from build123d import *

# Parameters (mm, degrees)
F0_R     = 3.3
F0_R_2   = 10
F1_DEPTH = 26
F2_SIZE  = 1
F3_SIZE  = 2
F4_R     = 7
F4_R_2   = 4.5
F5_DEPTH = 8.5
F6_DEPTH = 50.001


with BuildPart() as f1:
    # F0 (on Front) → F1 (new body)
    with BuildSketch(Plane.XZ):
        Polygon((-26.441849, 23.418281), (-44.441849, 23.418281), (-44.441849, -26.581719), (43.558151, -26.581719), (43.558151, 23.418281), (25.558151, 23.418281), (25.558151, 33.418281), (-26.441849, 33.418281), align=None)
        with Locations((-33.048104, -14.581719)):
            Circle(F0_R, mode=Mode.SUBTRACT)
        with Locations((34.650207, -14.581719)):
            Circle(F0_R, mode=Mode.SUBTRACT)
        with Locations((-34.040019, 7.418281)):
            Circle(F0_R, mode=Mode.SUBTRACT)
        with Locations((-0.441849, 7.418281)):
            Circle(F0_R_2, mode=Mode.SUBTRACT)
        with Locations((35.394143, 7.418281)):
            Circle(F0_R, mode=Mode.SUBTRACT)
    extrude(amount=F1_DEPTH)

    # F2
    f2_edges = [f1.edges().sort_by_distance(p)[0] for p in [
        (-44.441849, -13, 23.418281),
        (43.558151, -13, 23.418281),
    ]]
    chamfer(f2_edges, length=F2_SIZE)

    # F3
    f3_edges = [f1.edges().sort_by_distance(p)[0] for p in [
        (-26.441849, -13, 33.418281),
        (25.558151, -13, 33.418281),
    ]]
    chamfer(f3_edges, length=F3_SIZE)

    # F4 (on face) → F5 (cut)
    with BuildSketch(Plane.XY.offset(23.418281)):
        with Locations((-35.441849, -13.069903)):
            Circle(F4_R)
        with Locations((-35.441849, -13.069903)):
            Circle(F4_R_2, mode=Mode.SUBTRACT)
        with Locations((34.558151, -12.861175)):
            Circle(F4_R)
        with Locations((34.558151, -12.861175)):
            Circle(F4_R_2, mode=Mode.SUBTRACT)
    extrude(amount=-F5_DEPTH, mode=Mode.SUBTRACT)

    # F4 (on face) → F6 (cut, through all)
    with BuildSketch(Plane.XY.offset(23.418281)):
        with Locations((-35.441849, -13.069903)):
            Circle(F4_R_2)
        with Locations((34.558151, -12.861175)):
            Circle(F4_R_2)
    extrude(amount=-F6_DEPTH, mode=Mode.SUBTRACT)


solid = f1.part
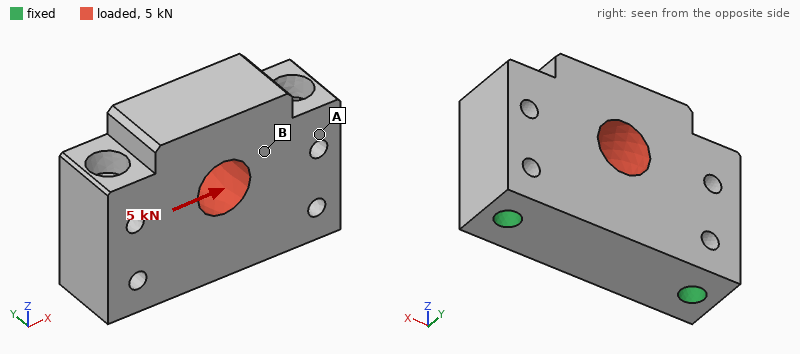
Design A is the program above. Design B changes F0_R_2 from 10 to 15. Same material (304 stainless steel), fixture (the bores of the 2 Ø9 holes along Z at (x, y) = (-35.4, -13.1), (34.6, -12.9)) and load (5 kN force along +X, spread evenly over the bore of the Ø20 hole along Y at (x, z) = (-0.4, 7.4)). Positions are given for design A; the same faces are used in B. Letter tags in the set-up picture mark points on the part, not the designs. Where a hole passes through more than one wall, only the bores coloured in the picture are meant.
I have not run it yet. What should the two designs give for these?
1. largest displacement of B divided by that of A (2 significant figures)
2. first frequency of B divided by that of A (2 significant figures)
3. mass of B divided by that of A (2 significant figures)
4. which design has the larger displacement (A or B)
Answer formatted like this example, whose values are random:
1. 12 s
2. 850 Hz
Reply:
1. 1.3
2. 1.0
3. 0.91
4. B
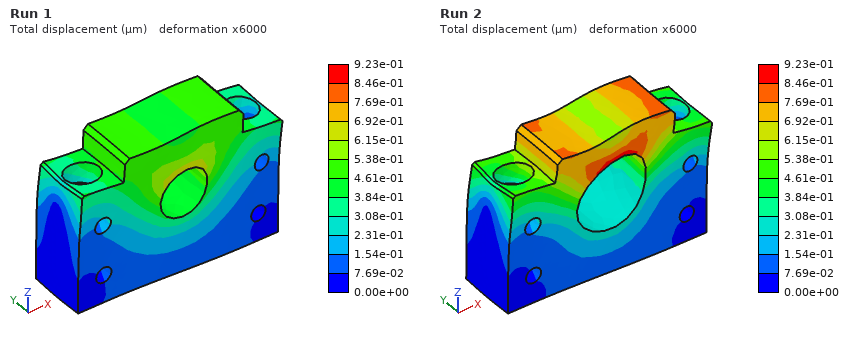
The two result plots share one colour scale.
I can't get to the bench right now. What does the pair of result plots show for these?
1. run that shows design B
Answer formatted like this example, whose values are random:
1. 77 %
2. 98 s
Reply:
1. Run 2
